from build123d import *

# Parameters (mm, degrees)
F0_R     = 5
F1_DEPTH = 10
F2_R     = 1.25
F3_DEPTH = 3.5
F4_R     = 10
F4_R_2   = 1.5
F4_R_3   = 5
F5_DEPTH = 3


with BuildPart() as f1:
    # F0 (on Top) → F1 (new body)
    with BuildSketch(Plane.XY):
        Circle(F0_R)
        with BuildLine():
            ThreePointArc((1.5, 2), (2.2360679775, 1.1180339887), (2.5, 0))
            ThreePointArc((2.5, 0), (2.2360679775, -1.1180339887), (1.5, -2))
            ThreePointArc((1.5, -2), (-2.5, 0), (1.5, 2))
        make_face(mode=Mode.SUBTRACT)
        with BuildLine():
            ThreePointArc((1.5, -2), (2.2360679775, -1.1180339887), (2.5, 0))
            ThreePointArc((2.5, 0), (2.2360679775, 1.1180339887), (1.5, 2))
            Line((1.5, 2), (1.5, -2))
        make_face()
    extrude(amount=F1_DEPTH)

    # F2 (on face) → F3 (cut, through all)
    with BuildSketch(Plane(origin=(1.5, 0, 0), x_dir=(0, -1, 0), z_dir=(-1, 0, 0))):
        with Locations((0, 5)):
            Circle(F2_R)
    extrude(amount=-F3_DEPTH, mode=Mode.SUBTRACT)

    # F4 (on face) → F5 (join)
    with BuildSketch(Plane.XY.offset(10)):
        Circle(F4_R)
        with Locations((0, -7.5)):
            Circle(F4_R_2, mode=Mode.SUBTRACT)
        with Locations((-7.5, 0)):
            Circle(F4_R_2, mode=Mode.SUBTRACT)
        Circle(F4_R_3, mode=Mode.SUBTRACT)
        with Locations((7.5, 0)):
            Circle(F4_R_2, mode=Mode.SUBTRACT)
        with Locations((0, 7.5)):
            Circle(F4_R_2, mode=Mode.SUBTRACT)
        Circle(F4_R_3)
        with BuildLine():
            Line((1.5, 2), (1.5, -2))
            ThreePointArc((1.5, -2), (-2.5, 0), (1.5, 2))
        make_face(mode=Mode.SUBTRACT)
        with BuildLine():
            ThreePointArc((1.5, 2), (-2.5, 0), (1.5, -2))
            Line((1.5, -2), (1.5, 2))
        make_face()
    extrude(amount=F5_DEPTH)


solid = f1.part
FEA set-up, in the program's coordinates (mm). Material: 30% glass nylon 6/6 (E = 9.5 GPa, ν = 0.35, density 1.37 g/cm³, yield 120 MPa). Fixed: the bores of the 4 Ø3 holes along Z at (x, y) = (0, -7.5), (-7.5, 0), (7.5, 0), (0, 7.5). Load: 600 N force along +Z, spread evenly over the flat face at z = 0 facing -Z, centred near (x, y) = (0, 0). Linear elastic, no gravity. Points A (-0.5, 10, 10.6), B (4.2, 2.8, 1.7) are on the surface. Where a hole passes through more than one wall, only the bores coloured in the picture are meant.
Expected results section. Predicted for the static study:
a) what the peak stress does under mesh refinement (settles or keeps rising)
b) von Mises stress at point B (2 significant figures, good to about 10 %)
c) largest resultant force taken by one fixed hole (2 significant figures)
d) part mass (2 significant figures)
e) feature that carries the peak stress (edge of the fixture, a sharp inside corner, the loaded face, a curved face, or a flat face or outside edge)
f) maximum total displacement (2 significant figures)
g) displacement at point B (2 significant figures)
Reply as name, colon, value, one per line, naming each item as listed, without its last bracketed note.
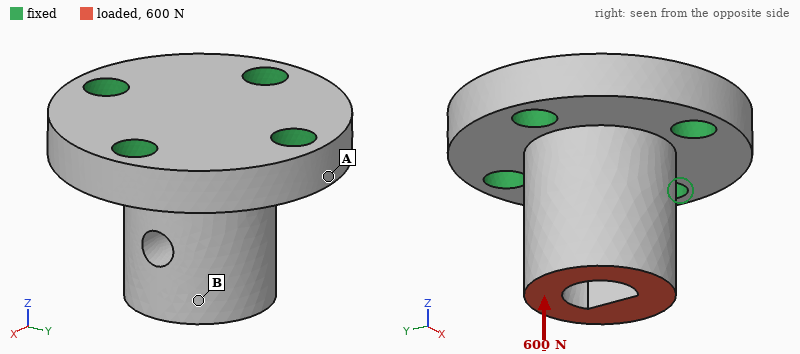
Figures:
what the peak stress does under mesh refinement: keeps rising
von Mises stress at point B: 12 MPa
largest resultant force taken by one fixed hole: 160 N
part mass: 2.0 g
feature that carries the peak stress: edge of the fixture
maximum total displacement: 23 µm
displacement at point B: 19 µm
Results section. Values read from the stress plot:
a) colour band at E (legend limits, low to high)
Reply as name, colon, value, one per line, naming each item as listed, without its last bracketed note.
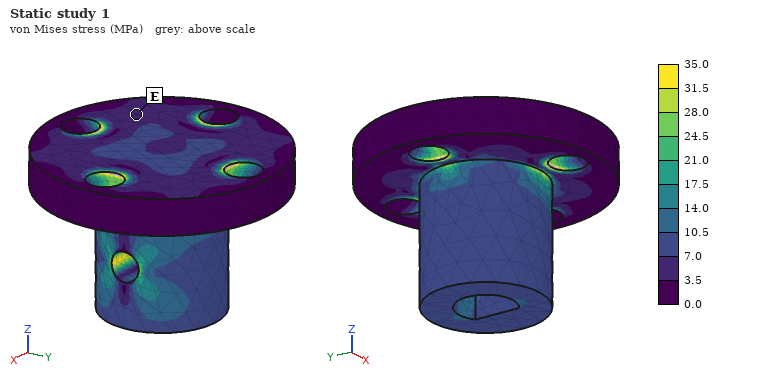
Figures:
colour band at E: 3.5 to 7.0 MPa
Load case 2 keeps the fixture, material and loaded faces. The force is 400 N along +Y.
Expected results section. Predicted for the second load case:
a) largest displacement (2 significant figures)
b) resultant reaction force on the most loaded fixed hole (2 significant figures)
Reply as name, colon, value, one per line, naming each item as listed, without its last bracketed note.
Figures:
largest displacement: 0.11 mm
resultant reaction force on the most loaded fixed hole: 370 N
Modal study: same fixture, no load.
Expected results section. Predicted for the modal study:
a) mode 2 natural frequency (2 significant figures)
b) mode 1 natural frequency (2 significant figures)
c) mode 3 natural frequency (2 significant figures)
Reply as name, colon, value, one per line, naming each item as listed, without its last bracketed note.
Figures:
mode 2 natural frequency: 18 kHz
mode 1 natural frequency: 18 kHz
mode 3 natural frequency: 35 kHz
